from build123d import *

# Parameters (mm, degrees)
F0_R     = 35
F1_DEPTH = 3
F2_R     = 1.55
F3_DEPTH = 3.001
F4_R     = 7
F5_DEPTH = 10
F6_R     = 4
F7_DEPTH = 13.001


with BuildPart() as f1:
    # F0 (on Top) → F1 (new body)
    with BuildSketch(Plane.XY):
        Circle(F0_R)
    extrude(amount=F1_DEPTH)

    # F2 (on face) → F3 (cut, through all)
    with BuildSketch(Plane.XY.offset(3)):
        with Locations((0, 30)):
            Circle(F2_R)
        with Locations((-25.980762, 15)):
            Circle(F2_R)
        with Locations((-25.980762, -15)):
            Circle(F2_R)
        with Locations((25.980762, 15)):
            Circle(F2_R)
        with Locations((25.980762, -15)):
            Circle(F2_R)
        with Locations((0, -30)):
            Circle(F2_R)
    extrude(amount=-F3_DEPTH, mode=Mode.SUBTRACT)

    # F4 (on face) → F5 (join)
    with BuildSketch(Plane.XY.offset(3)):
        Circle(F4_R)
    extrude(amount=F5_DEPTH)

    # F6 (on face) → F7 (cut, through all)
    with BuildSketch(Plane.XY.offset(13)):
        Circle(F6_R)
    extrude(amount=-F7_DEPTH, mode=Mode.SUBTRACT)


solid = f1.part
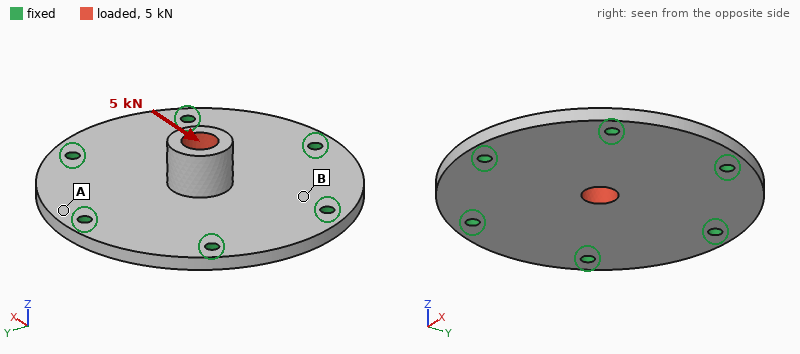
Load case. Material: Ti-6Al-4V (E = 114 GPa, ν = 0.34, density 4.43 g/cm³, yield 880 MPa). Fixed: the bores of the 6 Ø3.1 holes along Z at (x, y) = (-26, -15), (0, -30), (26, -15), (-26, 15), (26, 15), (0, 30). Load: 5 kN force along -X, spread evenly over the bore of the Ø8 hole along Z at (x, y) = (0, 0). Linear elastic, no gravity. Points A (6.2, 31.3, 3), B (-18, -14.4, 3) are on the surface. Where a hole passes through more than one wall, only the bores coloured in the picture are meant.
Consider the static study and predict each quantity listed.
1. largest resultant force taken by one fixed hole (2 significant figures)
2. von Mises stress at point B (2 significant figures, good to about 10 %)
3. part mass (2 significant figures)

1.2 kN
43 MPa
54 g
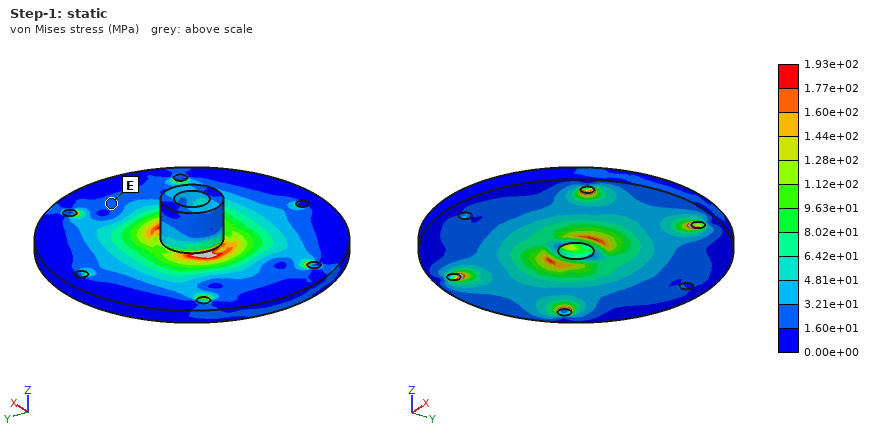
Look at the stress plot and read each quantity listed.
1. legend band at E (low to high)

1.60e+01 to 3.21e+01 MPa
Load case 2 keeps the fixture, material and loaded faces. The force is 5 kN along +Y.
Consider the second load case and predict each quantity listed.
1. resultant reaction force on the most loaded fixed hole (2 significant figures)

1.3 kN
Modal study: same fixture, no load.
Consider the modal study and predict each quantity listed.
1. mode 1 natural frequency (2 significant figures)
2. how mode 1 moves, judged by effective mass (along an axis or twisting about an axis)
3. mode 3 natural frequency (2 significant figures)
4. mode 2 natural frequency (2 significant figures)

6200 Hz
along Z
12 kHz
12 kHz
